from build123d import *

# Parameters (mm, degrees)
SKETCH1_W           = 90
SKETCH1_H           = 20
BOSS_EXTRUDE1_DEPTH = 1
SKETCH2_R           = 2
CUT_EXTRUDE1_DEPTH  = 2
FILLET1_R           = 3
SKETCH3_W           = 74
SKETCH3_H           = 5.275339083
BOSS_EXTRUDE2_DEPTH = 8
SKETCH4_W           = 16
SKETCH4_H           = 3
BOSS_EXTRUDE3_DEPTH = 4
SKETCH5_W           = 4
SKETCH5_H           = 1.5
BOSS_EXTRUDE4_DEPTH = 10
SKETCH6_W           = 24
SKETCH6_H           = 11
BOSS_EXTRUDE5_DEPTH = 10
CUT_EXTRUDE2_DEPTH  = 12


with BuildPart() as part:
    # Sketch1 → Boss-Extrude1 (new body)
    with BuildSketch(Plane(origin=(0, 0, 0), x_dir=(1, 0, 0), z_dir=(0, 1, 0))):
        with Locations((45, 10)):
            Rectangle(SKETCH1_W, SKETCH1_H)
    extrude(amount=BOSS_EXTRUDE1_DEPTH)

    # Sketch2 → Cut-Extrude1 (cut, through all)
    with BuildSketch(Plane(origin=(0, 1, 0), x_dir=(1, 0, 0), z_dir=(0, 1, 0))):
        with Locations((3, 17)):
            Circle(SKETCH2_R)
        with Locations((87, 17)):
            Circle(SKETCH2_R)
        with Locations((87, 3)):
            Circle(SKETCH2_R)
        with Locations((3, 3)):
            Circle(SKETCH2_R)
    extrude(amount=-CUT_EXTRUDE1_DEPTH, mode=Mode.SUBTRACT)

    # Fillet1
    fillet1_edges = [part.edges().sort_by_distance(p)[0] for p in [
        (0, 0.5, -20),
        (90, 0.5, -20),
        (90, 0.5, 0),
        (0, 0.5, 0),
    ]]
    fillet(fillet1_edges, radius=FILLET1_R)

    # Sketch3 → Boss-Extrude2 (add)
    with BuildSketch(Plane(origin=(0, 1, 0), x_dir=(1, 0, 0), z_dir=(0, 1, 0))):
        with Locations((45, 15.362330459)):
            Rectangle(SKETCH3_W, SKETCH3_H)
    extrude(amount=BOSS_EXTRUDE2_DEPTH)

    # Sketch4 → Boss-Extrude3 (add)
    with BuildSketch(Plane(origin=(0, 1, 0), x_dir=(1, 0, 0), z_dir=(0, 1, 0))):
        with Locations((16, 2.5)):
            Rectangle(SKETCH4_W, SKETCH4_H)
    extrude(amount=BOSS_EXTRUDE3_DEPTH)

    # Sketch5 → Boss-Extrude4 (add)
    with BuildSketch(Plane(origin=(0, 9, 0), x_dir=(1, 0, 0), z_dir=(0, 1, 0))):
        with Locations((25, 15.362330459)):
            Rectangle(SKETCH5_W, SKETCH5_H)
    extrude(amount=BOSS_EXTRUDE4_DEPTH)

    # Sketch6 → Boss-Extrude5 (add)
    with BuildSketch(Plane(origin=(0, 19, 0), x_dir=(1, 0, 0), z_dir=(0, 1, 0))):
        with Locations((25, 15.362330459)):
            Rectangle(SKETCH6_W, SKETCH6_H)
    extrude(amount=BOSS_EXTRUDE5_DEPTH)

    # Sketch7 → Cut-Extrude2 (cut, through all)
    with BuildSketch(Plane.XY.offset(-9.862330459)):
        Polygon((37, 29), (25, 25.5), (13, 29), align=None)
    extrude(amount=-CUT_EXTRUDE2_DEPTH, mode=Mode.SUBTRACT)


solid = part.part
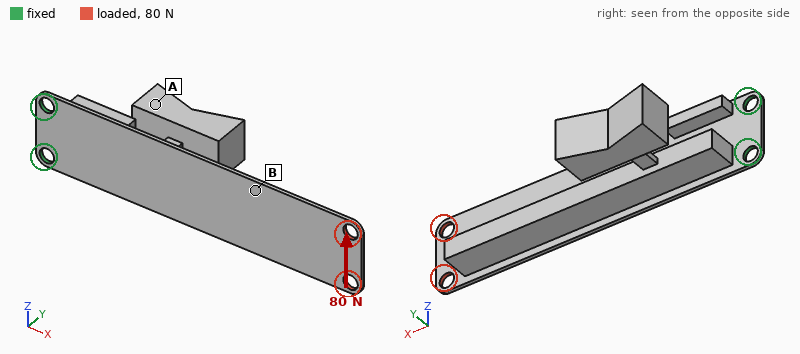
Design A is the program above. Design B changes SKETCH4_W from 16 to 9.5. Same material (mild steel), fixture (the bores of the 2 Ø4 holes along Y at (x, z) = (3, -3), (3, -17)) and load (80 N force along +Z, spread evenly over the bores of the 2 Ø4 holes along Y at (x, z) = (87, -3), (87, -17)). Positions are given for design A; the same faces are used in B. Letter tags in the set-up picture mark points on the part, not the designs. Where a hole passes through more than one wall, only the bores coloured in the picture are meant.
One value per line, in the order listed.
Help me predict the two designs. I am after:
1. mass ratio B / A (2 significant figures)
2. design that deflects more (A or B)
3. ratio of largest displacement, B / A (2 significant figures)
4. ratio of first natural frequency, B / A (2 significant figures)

0.99
B
1.1
0.94
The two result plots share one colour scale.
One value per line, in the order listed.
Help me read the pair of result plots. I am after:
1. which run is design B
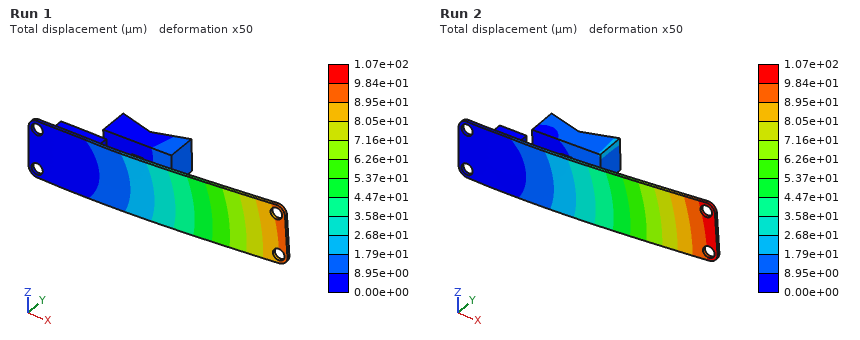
Run 2
